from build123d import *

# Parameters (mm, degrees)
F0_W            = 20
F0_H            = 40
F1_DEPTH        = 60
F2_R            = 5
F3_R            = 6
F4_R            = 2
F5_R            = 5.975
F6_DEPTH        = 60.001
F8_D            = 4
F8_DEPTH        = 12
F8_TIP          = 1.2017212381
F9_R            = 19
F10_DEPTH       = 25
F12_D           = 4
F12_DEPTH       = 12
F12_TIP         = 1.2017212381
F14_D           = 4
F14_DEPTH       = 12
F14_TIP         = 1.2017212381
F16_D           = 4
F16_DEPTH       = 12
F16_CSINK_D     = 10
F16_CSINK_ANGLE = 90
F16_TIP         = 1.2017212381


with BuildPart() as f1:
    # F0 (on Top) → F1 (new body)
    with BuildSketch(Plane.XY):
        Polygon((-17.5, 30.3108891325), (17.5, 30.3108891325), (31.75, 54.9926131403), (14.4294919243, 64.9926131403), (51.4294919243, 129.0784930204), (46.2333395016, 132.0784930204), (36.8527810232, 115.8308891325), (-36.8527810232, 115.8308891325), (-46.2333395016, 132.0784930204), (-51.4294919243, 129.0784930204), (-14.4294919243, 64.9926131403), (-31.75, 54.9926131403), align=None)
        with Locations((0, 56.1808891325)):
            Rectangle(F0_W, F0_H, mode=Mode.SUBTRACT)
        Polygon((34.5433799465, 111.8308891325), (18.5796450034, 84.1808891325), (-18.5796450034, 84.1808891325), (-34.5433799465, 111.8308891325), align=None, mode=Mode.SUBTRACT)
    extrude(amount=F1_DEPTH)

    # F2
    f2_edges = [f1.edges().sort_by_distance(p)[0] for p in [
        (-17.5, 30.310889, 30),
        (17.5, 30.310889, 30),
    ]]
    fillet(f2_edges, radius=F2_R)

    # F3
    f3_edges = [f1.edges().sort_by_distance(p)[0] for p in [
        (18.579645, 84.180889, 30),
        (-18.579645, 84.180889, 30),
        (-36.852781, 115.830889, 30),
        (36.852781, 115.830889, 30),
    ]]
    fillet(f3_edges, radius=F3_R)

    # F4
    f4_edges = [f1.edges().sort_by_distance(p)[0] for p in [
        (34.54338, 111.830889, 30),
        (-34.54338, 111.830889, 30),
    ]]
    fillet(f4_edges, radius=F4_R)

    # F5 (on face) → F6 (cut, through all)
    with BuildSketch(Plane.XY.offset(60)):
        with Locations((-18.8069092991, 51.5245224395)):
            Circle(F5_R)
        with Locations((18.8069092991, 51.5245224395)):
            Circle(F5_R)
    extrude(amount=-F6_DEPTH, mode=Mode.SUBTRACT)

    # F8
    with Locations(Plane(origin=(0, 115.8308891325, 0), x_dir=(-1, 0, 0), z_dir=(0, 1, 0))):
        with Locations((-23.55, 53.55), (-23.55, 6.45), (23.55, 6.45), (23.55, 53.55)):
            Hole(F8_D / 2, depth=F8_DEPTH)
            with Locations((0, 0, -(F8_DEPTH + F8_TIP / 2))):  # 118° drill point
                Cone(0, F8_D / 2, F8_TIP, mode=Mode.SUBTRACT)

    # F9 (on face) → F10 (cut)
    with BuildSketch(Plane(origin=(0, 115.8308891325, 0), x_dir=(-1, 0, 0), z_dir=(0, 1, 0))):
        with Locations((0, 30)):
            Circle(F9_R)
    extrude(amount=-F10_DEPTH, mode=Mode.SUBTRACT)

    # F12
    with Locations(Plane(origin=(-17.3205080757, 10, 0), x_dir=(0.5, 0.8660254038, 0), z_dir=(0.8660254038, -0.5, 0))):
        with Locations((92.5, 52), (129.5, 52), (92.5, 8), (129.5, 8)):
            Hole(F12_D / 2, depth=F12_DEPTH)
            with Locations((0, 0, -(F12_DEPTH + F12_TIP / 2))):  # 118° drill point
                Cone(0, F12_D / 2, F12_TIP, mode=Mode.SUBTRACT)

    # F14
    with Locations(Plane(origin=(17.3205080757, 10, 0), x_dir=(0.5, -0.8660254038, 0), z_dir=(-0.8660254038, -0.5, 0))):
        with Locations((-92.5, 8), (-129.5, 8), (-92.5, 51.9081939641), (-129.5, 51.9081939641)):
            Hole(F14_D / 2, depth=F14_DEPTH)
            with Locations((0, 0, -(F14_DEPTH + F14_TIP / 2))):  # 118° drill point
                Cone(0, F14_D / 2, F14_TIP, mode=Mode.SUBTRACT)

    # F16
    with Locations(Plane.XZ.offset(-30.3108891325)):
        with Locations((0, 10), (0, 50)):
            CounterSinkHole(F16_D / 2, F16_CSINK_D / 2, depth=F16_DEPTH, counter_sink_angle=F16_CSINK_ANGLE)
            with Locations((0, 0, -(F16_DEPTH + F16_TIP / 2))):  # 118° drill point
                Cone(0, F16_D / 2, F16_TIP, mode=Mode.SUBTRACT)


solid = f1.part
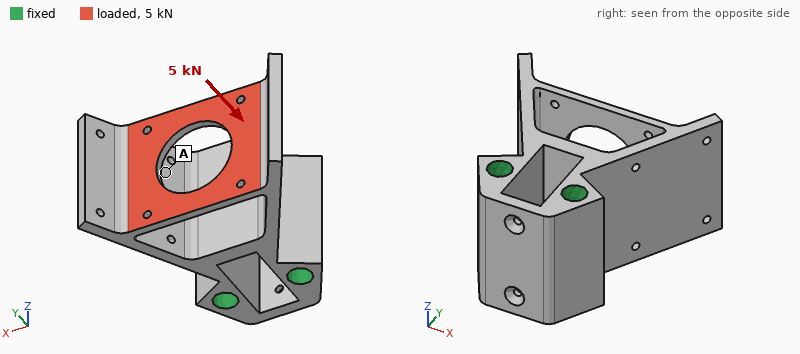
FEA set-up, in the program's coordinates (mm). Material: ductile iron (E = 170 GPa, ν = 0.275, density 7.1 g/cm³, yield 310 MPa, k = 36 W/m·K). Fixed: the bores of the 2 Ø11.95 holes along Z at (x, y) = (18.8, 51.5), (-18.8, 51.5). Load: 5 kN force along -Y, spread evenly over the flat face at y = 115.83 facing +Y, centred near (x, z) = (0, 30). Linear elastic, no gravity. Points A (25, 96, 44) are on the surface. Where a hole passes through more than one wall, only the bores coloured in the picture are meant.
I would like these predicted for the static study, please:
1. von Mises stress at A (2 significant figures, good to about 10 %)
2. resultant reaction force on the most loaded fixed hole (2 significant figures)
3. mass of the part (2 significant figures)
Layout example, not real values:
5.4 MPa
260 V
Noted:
25 MPa
3.0 kN
960 g
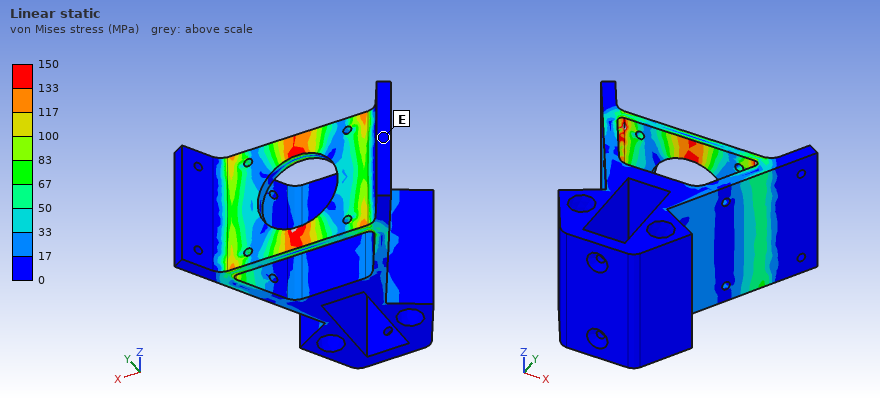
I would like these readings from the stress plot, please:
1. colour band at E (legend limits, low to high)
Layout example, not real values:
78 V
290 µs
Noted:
0 to 17 MPa
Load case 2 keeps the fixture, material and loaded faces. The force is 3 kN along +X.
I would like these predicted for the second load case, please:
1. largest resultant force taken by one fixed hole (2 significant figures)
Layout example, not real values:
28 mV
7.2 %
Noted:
5.1 kN
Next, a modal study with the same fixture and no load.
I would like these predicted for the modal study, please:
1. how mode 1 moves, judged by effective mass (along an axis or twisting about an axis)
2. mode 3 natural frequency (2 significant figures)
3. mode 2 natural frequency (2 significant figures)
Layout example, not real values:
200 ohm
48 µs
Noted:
along X
4000 Hz
3900 Hz
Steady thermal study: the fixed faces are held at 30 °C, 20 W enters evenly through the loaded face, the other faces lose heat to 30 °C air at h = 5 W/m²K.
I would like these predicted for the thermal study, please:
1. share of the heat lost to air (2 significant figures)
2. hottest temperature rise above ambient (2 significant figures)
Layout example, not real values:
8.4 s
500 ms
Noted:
19 %
59 K
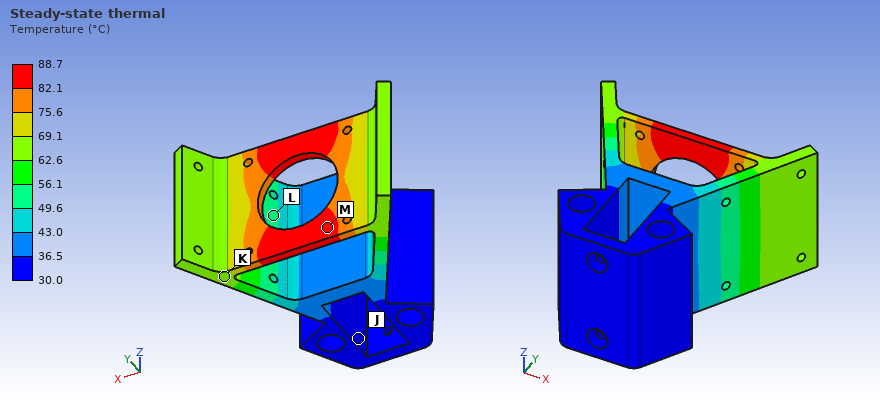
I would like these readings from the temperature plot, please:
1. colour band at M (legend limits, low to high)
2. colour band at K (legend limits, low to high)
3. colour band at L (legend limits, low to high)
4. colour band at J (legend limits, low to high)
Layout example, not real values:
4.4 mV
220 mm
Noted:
82.1 to 88.7 °C
62.6 to 69.1 °C
49.6 to 56.1 °C
30.0 to 36.5 °C
